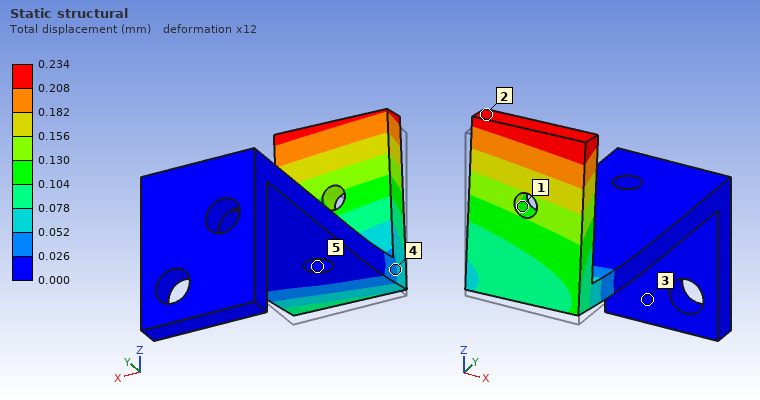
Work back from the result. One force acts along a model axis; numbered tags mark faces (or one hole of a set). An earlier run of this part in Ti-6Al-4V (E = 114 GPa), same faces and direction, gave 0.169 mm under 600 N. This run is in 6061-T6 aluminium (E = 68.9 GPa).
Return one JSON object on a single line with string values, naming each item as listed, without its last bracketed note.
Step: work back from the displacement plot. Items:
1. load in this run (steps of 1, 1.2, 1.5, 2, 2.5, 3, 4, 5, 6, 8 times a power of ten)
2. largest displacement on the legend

{"load in this run": "500 N", "largest displacement on the legend": "0.234 mm"}
